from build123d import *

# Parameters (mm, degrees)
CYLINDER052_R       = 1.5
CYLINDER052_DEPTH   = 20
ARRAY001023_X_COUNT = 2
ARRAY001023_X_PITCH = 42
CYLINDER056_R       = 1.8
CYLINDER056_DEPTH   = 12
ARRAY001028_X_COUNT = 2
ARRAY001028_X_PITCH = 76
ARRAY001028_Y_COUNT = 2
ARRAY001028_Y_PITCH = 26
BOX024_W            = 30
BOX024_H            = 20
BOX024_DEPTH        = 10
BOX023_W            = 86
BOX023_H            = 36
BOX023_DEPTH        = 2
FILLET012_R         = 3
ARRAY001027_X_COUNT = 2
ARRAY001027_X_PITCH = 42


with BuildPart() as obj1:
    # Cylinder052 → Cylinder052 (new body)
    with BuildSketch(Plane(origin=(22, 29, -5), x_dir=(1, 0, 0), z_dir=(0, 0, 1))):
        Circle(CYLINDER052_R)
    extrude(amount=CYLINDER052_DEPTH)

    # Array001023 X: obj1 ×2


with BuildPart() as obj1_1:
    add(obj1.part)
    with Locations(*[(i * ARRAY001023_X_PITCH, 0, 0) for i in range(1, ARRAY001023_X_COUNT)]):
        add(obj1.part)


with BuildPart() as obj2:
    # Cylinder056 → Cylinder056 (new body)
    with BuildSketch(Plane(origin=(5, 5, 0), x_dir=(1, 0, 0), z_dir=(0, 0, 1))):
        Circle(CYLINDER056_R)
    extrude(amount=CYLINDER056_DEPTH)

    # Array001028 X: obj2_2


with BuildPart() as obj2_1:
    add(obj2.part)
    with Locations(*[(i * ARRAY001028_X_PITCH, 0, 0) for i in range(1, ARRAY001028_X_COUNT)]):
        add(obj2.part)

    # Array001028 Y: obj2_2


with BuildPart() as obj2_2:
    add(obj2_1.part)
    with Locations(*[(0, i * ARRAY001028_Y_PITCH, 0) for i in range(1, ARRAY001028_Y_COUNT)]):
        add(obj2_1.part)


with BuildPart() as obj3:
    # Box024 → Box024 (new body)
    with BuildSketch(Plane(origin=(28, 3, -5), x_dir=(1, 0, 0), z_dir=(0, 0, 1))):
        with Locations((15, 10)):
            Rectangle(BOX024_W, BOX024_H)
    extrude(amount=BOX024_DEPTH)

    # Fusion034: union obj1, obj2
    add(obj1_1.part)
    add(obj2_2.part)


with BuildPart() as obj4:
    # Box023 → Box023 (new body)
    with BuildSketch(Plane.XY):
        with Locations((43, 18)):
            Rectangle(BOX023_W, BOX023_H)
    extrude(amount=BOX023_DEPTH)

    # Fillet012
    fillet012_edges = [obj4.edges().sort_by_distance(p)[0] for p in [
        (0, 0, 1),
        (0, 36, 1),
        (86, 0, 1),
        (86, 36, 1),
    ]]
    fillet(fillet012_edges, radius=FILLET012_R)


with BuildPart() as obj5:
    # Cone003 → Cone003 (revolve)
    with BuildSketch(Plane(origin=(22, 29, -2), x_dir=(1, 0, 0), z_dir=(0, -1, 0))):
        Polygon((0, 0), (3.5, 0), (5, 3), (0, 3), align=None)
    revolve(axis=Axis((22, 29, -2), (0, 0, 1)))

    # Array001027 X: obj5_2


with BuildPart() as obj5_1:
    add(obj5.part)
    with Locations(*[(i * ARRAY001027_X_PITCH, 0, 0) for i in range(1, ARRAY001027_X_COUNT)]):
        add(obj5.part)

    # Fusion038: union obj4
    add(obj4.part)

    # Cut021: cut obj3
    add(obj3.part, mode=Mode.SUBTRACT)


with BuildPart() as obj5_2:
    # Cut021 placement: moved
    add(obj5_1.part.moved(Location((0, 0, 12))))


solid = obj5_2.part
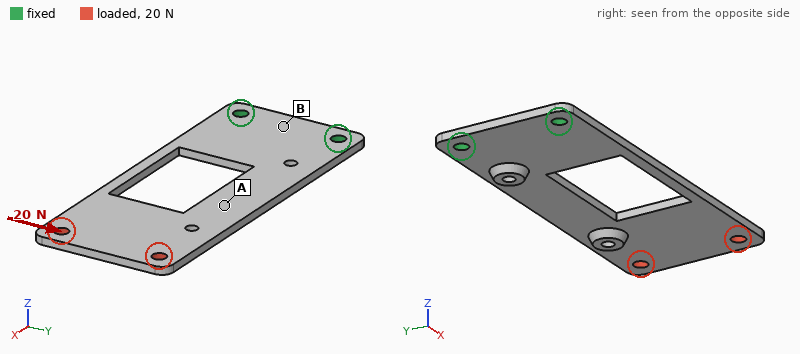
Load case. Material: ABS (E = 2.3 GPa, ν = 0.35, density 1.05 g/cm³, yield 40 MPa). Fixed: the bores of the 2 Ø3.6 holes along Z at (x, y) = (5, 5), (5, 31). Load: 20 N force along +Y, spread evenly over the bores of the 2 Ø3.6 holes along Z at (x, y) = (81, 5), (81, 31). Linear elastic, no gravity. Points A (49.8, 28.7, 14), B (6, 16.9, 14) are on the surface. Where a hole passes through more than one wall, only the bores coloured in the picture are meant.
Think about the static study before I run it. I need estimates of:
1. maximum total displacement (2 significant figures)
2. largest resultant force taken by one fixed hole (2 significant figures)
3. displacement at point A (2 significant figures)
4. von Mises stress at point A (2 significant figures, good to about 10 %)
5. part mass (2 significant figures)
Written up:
0.47 mm
58 N
0.23 mm
2.2 MPa
5.3 g
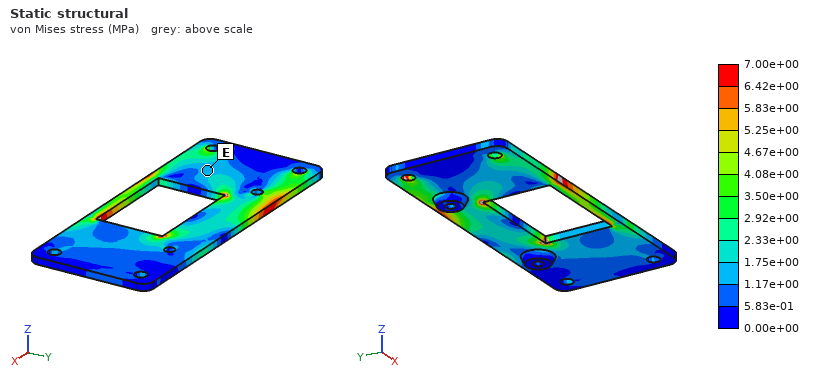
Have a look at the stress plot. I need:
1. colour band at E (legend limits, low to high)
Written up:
1.17e+00 to 1.75e+00 MPa
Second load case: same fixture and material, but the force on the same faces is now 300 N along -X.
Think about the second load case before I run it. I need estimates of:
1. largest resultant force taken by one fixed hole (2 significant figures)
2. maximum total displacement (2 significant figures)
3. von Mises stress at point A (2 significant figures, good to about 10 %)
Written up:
150 N
0.72 mm
7.6 MPa
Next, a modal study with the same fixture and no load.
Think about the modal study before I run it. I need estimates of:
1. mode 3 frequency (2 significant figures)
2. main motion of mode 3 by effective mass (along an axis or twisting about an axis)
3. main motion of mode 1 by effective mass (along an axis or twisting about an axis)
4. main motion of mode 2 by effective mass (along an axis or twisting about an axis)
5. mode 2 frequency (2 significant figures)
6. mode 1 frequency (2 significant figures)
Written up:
460 Hz
along Z
along Z
twisting about X
290 Hz
66 Hz
